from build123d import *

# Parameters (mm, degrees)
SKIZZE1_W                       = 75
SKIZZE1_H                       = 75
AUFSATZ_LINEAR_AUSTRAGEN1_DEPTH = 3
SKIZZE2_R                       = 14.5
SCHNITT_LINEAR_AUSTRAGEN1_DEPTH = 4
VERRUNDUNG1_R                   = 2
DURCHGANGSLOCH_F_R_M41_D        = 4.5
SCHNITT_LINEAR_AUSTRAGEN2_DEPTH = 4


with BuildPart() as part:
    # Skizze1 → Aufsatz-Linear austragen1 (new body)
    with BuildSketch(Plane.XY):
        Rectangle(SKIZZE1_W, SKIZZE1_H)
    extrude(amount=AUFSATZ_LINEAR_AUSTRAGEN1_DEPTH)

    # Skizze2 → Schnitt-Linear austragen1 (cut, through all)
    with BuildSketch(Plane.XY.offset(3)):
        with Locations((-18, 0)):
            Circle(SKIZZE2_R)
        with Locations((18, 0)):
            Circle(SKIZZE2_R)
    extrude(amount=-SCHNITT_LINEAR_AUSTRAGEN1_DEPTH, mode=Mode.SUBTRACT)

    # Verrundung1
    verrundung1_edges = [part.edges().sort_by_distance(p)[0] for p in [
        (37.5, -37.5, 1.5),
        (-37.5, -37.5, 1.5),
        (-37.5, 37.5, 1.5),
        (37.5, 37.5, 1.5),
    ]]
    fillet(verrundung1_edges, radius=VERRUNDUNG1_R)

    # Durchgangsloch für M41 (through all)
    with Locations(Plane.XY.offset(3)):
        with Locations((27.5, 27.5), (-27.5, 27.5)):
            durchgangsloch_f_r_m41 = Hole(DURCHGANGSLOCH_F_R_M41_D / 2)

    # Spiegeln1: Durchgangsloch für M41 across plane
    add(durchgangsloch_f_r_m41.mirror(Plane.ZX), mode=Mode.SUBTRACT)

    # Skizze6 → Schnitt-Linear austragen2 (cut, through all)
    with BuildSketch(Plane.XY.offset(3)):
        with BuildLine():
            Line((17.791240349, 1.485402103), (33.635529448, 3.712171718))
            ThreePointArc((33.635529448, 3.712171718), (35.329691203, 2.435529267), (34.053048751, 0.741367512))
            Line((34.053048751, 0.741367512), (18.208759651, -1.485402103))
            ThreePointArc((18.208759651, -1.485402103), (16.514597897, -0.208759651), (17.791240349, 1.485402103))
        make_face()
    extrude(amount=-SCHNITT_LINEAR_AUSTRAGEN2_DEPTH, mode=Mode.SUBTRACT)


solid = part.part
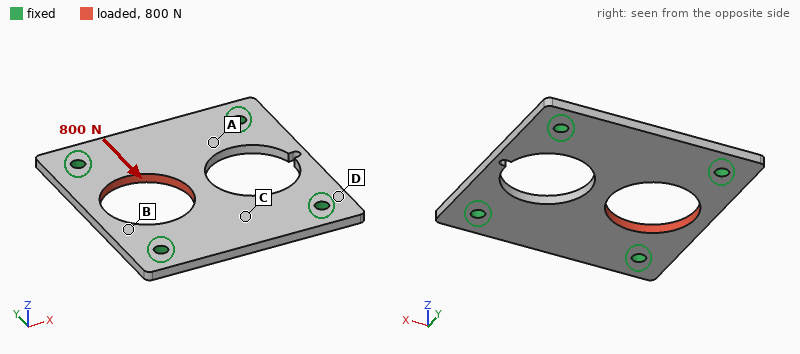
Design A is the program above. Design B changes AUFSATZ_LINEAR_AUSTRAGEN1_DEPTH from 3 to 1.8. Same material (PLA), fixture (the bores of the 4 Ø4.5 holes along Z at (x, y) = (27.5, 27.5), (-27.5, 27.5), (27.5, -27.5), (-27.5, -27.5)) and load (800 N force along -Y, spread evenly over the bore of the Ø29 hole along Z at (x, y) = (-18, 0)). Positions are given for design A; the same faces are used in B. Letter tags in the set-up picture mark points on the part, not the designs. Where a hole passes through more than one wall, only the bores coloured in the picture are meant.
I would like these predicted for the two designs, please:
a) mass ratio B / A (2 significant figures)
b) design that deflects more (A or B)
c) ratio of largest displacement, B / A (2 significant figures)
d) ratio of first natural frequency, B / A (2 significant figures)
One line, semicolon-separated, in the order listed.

0.60; B; 1.7; 0.62
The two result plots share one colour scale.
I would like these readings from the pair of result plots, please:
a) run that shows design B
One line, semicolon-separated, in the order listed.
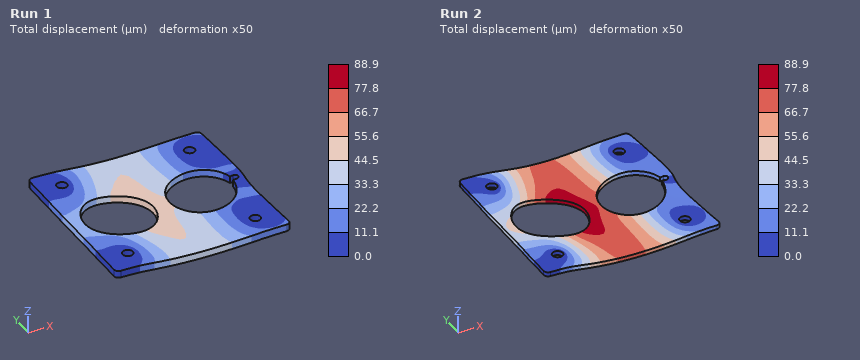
Run 2
